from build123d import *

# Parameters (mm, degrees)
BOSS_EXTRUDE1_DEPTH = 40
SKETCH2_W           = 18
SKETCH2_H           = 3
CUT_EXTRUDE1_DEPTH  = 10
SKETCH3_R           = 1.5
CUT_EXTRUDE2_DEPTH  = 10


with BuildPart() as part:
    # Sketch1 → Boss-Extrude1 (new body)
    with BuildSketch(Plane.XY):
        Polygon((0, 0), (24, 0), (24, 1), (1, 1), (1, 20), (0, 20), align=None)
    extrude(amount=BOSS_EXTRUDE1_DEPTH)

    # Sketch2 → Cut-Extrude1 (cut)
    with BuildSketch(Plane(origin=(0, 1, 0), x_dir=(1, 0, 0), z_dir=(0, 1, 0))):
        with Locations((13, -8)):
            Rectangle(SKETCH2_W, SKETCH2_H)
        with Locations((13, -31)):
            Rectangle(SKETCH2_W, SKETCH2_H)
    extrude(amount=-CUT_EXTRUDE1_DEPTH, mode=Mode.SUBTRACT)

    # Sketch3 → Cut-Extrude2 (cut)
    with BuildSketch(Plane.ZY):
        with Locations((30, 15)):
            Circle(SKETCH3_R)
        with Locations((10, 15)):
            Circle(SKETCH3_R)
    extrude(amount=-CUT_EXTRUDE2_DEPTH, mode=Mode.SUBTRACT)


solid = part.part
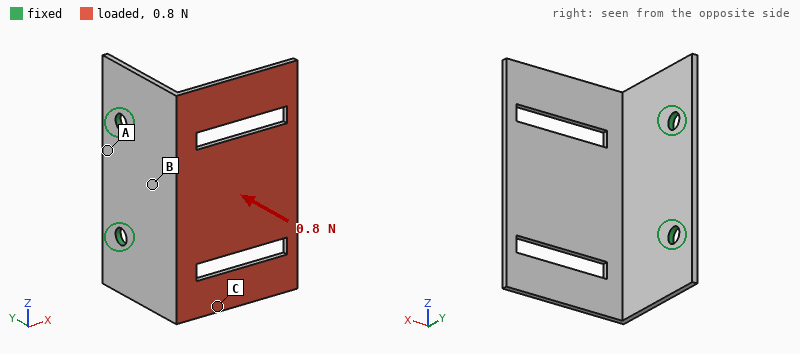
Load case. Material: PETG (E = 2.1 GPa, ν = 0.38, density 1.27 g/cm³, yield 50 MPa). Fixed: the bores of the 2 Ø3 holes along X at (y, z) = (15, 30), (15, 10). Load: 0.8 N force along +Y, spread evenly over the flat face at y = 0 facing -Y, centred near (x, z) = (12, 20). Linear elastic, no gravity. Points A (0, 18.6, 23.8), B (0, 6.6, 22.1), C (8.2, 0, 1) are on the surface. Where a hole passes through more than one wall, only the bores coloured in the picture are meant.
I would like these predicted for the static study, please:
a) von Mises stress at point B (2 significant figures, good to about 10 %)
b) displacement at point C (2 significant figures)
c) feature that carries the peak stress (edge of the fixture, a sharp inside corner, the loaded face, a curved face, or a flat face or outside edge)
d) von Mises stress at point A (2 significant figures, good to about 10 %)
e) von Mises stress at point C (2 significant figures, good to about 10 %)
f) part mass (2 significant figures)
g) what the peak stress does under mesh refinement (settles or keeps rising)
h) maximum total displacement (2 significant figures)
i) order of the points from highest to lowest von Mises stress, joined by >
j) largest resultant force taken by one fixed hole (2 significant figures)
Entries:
1.2 MPa
0.21 mm
edge of the fixture
0.29 MPa
0.73 MPa
2.0 g
keeps rising
0.60 mm
B > C > A
0.41 N
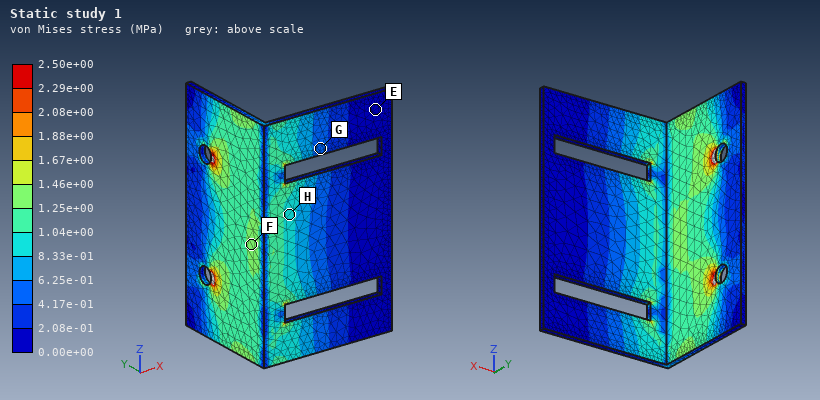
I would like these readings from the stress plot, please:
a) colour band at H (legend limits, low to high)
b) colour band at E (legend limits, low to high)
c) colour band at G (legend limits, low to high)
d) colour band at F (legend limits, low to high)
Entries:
8.33e-01 to 1.04e+00 MPa
0.00e+00 to 2.08e-01 MPa
4.17e-01 to 6.25e-01 MPa
1.25e+00 to 1.46e+00 MPa
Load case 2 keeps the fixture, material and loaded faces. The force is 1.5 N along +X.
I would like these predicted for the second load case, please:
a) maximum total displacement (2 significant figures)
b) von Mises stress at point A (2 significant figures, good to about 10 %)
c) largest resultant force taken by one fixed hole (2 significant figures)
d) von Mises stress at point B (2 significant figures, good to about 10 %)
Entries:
0.59 mm
0.63 MPa
0.75 N
1.3 MPa
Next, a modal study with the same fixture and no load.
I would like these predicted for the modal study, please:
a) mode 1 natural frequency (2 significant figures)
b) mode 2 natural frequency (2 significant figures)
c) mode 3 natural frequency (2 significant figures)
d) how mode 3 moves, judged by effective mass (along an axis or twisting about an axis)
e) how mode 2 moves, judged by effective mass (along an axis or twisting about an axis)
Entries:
200 Hz
360 Hz
590 Hz
along X
along Z
